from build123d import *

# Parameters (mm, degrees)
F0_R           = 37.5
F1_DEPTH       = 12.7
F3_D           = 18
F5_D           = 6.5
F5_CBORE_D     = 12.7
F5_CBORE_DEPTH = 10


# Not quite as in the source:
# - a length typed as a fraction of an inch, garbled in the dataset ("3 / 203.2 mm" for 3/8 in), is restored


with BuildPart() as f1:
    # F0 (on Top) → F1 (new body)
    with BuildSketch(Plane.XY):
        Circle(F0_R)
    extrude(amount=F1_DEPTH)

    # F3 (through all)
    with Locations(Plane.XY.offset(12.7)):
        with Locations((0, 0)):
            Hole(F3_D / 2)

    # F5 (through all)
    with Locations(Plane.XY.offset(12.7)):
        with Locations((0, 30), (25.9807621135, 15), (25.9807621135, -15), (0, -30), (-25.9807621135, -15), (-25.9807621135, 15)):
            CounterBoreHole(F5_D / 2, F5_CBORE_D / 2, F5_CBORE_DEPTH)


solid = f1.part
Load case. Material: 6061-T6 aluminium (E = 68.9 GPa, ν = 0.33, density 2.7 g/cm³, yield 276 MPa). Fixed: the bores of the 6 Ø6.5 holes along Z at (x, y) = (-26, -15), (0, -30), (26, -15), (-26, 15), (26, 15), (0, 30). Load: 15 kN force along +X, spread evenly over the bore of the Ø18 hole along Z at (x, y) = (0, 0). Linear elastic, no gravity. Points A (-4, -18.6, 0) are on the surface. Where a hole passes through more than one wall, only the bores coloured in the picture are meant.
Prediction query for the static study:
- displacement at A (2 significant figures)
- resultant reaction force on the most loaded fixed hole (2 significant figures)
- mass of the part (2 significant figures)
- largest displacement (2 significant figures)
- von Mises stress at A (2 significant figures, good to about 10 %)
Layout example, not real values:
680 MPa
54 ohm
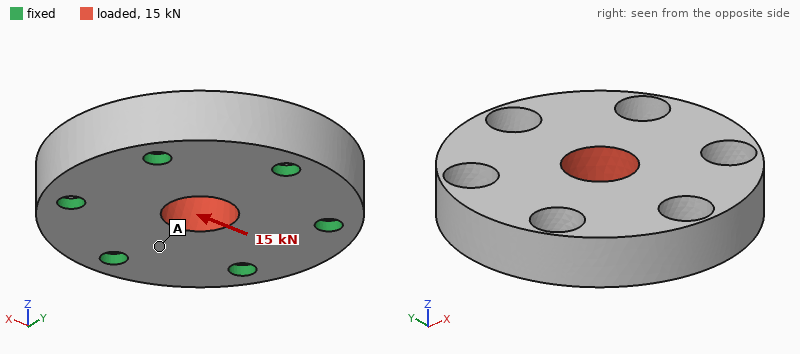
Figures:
6.5 µm
3.0 kN
120 g
15 µm
17 MPa
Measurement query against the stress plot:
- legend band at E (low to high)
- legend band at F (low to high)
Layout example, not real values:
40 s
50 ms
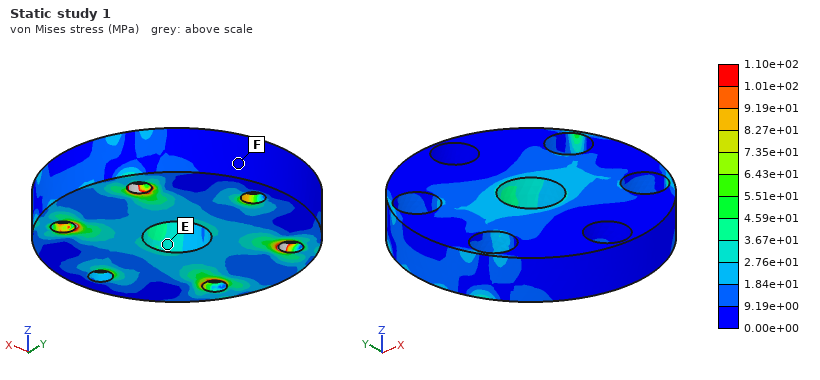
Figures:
2.76e+01 to 3.67e+01 MPa
0.00e+00 to 9.19e+00 MPa
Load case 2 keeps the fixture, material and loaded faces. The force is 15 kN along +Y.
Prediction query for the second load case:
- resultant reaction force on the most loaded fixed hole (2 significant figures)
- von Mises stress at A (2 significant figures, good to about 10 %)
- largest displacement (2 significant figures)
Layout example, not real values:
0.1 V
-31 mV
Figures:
3.3 kN
31 MPa
15 µm
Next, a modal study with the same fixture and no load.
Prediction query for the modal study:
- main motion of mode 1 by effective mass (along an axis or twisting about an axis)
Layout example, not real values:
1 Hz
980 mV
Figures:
along Z
